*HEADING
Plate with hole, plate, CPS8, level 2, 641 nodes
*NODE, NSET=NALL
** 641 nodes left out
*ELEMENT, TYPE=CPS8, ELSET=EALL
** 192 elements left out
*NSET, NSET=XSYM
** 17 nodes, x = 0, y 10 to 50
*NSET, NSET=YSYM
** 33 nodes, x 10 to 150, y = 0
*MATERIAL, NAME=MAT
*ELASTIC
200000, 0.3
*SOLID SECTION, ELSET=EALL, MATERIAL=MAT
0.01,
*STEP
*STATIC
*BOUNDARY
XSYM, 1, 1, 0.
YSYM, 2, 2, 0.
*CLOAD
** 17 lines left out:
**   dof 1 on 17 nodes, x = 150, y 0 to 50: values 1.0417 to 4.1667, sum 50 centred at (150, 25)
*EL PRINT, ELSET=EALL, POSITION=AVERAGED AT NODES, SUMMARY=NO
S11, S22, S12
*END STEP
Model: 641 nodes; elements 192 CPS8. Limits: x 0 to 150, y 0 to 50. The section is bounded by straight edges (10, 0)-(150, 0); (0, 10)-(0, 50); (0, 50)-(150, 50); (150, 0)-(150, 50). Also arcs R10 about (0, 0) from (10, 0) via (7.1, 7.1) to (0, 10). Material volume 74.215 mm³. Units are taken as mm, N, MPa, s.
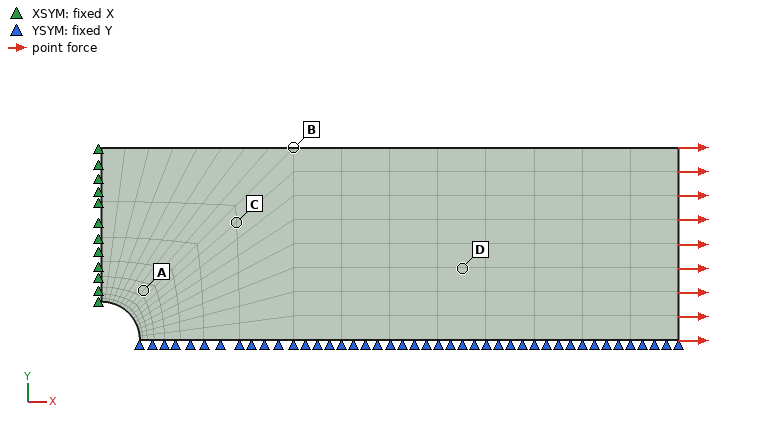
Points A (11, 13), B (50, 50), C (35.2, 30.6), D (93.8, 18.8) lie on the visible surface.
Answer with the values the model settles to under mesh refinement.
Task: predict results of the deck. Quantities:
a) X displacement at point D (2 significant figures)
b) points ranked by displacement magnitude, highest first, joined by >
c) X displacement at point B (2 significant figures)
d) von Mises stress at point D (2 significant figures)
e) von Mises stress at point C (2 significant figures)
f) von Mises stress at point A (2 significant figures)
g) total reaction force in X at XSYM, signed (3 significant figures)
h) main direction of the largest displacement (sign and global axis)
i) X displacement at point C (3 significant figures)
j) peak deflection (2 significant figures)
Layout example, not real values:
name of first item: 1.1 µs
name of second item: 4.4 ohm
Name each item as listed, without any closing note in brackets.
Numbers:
X displacement at point D: 0.049 mm
points ranked by displacement magnitude, highest first, joined by >: D > B > C > A
X displacement at point B: 0.026 mm
von Mises stress at point D: 99 MPa
von Mises stress at point C: 110 MPa
von Mises stress at point A: 140 MPa
total reaction force in X at XSYM, signed: -50.0 N
main direction of the largest displacement: +X
X displacement at point C: 0.0195 mm
peak deflection: 0.079 mm
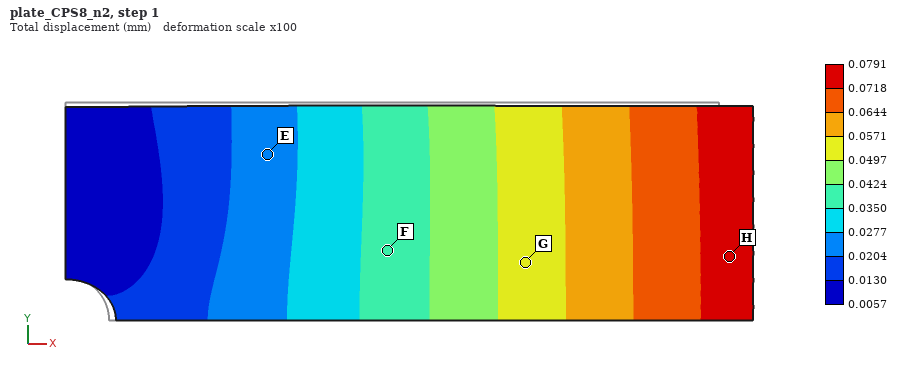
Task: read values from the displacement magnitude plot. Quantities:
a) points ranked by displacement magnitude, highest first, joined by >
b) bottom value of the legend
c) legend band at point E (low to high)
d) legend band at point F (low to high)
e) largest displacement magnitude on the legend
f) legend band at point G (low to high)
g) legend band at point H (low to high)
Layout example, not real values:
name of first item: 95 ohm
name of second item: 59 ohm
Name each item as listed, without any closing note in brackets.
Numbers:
points ranked by displacement magnitude, highest first, joined by >: H > G > F > E
bottom value of the legend: 0.0057 mm
legend band at point E: 0.0204 to 0.0277 mm
legend band at point F: 0.0350 to 0.0424 mm
largest displacement magnitude on the legend: 0.0791 mm
legend band at point G: 0.0497 to 0.0571 mm
legend band at point H: 0.0718 to 0.0791 mm
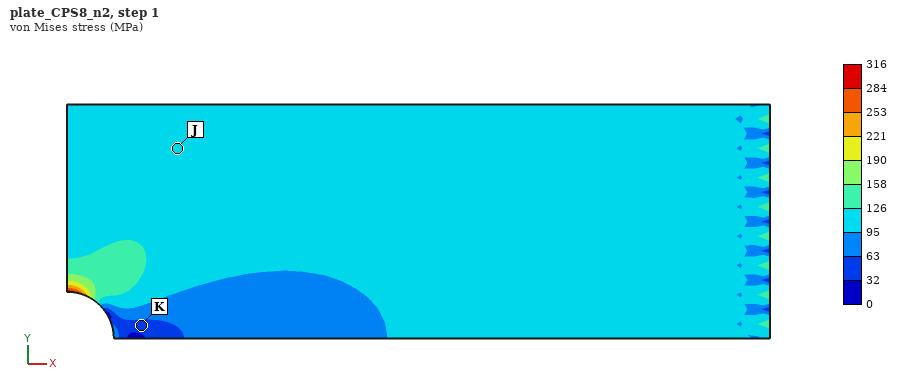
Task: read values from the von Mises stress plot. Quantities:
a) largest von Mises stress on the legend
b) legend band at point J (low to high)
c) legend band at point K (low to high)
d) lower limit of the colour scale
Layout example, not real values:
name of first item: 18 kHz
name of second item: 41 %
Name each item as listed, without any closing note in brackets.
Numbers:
largest von Mises stress on the legend: 316 MPa
legend band at point J: 95 to 126 MPa
legend band at point K: 32 to 63 MPa
lower limit of the colour scale: 0 MPa
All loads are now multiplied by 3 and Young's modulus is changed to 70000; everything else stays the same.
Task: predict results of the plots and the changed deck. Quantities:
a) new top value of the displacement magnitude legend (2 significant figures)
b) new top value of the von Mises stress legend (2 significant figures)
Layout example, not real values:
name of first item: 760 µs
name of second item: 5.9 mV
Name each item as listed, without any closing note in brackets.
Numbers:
new top value of the displacement magnitude legend: 0.68 mm
new top value of the von Mises stress legend: 950 MPa
